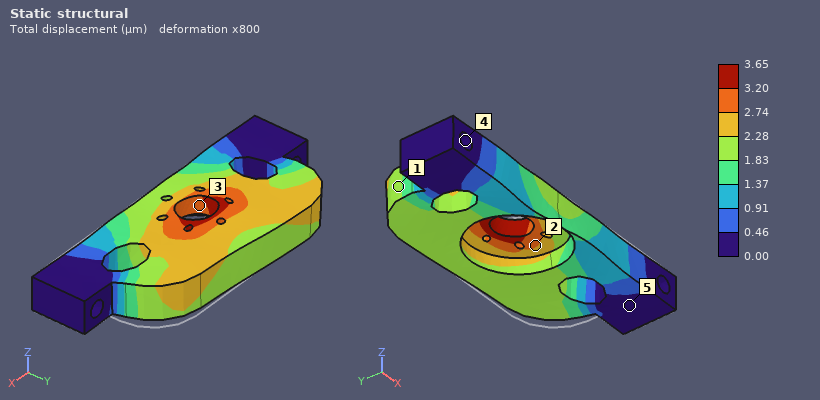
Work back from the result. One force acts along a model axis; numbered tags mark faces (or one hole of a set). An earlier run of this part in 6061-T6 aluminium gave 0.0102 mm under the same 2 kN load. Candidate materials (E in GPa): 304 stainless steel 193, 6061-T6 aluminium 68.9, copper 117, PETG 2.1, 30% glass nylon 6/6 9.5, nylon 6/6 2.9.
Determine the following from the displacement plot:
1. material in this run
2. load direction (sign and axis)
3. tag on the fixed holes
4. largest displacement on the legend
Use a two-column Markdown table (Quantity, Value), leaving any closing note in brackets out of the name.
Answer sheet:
| Quantity | Value |
|---|---|
| material in this run | 304 stainless steel |
| load direction | -X |
| tag on the fixed holes | 4 |
| largest displacement on the legend | 3.65 µm |
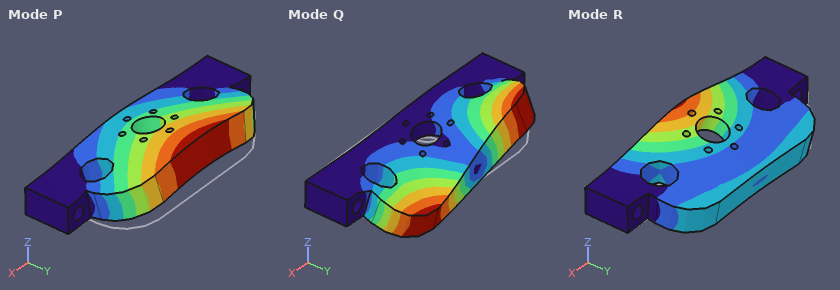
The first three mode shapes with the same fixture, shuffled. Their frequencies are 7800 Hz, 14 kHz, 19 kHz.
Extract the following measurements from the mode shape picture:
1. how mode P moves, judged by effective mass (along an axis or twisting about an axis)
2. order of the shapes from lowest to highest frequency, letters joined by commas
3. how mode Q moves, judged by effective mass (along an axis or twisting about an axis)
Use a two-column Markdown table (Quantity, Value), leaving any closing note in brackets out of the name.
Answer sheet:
| Quantity | Value |
|---|---|
| how mode P moves, judged by effective mass | along Z |
| order of the shapes from lowest to highest frequency, letters joined by commas | P, R, Q |
| how mode Q moves, judged by effective mass | twisting about Y |
